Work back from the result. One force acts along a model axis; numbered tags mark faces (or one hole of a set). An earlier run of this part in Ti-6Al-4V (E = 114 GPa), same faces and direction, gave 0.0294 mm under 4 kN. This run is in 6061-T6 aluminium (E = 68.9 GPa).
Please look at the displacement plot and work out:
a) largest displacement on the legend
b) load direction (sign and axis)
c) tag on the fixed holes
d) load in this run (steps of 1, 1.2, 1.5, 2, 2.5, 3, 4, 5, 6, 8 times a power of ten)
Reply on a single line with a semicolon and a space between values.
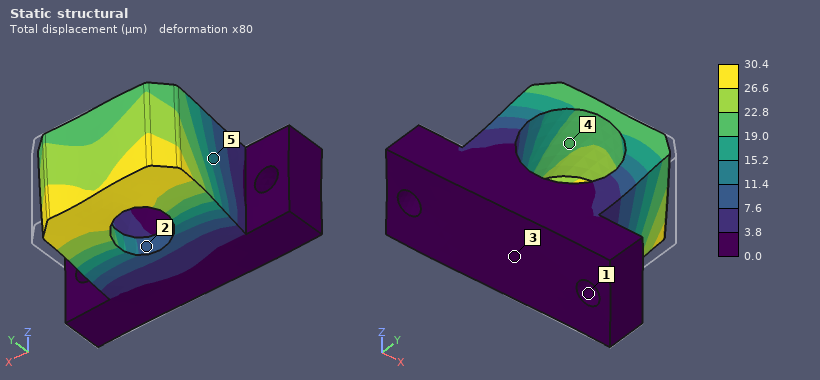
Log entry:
30.4 µm; -X; 1; 2.5 kN
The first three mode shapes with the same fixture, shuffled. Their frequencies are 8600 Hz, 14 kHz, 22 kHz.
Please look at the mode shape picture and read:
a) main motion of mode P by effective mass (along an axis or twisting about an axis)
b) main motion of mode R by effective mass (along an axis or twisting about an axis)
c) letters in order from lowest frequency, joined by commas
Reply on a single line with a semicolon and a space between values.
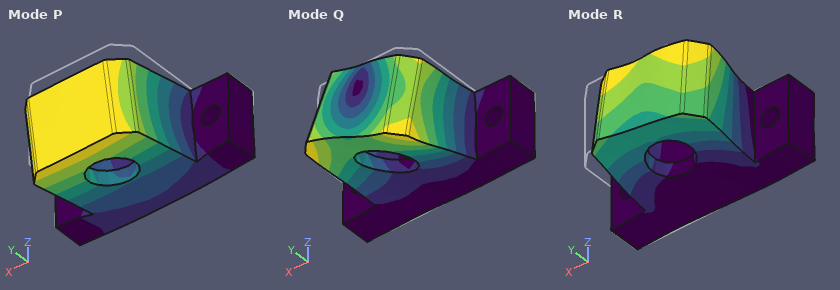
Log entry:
along Z; along X; P, R, Q
